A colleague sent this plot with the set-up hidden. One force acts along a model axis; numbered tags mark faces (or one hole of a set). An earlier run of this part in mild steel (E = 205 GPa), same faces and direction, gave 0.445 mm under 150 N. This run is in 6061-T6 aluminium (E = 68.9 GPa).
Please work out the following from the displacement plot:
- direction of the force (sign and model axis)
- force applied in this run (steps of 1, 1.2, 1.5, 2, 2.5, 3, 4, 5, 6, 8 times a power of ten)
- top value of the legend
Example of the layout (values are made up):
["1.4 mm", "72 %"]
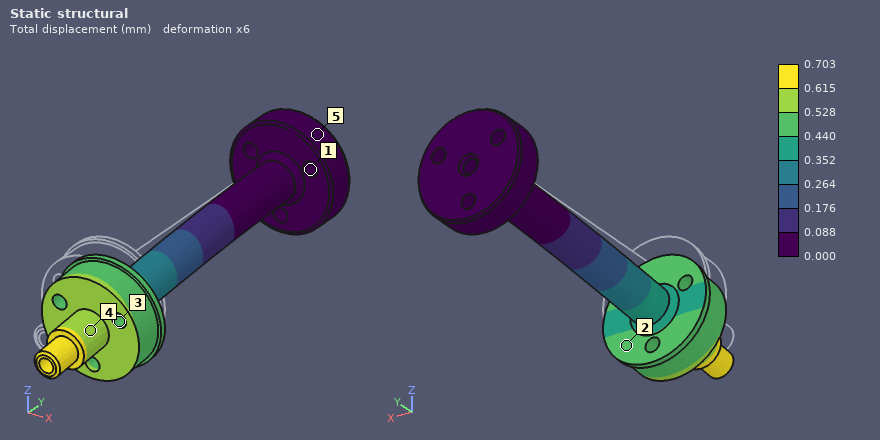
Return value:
["-Z", "80 N", "0.703 mm"]
